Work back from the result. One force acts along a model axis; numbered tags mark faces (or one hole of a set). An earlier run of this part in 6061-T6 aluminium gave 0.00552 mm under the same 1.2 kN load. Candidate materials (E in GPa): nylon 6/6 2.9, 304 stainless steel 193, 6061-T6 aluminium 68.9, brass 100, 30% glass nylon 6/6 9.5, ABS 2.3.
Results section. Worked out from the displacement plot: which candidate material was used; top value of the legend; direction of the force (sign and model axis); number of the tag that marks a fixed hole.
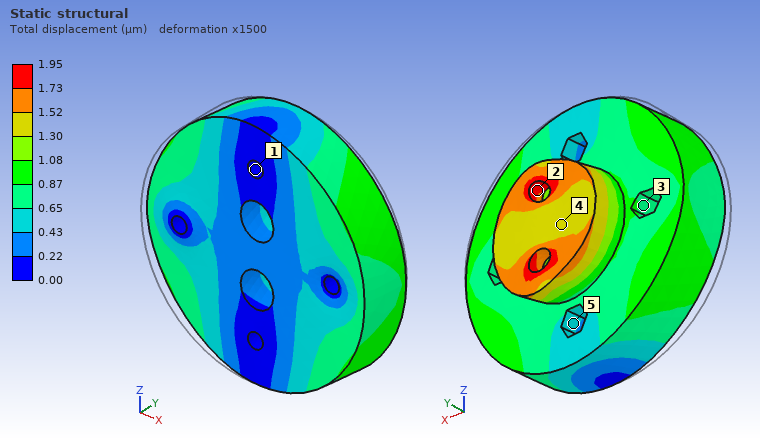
304 stainless steel
1.95 µm
+X
1
